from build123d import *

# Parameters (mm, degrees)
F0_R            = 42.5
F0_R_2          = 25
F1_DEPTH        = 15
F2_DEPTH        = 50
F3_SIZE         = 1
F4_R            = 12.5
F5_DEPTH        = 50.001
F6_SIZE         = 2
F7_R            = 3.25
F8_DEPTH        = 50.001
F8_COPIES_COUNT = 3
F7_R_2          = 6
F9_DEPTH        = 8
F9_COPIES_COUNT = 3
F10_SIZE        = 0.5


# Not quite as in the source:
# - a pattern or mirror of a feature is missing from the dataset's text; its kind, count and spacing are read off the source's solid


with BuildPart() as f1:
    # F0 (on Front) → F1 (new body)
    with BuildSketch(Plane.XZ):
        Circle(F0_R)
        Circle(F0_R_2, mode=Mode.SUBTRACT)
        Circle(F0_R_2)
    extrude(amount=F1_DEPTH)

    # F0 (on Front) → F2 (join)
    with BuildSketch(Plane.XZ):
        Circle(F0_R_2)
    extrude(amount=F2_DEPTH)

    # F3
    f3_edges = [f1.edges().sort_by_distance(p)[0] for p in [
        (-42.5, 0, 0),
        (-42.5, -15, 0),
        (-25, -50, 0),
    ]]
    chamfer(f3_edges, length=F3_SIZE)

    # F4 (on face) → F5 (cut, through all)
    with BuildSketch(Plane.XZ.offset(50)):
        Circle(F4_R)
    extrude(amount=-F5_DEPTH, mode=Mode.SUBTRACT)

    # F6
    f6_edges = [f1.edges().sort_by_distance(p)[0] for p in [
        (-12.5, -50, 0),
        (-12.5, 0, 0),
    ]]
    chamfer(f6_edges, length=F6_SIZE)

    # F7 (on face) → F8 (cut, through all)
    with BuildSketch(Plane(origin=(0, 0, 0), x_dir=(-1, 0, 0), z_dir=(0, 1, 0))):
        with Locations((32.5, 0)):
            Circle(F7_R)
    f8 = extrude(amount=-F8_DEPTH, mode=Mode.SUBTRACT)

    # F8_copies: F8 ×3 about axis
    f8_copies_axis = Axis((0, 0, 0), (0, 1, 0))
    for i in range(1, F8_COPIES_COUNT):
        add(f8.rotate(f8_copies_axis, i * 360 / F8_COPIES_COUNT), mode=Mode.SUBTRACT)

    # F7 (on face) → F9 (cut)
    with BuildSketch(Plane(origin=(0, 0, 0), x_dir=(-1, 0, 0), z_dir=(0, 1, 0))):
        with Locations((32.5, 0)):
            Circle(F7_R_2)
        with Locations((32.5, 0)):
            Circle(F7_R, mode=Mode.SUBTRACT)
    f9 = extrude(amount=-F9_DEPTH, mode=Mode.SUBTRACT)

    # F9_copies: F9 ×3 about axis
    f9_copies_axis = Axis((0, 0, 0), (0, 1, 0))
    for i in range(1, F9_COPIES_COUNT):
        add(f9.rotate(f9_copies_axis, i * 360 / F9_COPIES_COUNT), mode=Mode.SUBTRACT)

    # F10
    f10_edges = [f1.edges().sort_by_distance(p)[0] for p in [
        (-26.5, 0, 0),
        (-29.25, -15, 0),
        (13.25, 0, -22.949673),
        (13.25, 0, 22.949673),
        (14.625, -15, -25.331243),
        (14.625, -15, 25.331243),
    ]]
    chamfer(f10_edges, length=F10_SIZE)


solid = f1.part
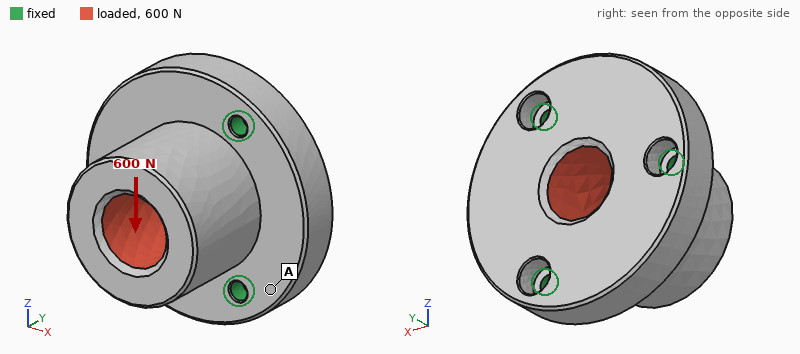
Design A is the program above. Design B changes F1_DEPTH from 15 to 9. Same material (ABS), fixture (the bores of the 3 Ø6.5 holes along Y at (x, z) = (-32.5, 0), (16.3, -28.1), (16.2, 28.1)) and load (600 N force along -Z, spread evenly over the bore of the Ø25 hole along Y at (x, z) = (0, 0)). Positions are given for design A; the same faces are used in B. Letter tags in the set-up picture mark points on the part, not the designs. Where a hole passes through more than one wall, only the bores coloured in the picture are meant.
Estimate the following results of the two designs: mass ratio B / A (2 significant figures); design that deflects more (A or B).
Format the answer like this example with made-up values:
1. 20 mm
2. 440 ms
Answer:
1. 0.83
2. B
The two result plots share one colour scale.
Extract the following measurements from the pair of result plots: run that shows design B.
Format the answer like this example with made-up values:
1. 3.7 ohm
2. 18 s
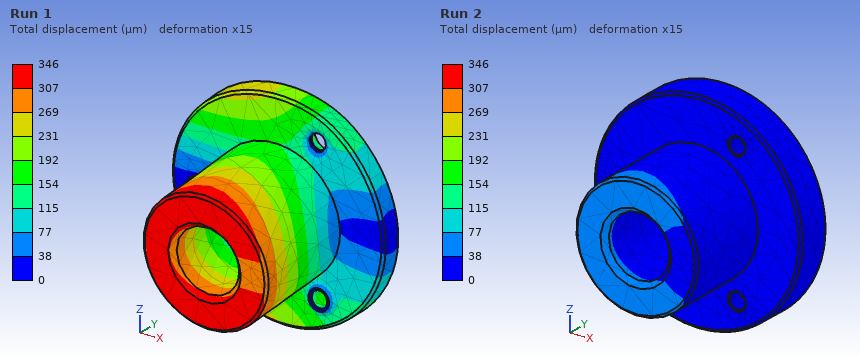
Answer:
1. Run 1
